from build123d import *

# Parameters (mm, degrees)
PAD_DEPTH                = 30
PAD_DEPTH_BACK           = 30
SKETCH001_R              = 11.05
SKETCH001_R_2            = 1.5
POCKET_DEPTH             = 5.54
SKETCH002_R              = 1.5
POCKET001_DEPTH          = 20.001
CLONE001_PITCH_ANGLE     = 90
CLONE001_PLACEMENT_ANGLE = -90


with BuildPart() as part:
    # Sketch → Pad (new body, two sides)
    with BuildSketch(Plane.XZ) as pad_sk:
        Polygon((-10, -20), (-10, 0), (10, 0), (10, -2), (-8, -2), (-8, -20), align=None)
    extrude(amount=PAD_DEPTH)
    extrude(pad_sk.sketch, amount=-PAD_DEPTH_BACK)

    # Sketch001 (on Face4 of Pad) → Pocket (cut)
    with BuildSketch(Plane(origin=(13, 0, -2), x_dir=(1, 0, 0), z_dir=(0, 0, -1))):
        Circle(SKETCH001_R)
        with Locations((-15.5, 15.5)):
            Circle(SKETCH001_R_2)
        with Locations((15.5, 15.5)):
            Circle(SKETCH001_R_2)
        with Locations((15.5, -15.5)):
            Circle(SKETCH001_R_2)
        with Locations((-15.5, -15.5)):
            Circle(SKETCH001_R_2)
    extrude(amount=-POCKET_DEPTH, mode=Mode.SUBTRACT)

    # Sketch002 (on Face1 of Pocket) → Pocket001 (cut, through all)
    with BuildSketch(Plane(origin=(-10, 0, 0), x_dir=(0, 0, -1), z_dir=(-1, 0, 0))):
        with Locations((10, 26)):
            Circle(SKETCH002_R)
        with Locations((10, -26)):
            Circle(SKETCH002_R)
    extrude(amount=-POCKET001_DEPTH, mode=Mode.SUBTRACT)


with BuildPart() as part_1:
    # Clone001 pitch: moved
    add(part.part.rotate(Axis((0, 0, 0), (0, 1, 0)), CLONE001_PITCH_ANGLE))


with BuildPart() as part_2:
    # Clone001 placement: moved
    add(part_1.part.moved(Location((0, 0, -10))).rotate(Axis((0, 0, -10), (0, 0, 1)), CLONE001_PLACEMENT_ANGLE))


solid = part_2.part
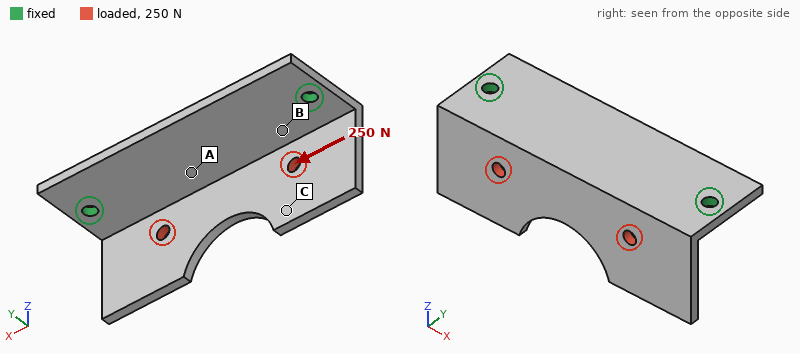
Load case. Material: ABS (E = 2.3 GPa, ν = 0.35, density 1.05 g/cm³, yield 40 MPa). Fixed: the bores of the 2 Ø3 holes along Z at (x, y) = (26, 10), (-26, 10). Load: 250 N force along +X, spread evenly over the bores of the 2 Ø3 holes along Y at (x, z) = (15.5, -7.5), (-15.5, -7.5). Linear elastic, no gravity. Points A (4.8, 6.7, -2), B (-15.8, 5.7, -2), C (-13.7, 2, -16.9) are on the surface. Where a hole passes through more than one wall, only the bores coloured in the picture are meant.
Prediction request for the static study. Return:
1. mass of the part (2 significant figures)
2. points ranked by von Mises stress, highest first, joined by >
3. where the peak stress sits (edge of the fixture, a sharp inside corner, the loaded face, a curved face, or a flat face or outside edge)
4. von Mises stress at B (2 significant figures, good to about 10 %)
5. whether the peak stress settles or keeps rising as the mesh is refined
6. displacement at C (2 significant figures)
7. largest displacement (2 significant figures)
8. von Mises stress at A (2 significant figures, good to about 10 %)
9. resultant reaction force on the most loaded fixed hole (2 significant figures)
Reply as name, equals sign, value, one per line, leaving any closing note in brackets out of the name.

mass of the part = 4.5 g
points ranked by von Mises stress, highest first, joined by > = B > A > C
where the peak stress sits = edge of the fixture
von Mises stress at B = 8.6 MPa
whether the peak stress settles or keeps rising as the mesh is refined = keeps rising
displacement at C = 0.36 mm
largest displacement = 0.66 mm
von Mises stress at A = 5.2 MPa
resultant reaction force on the most loaded fixed hole = 140 N
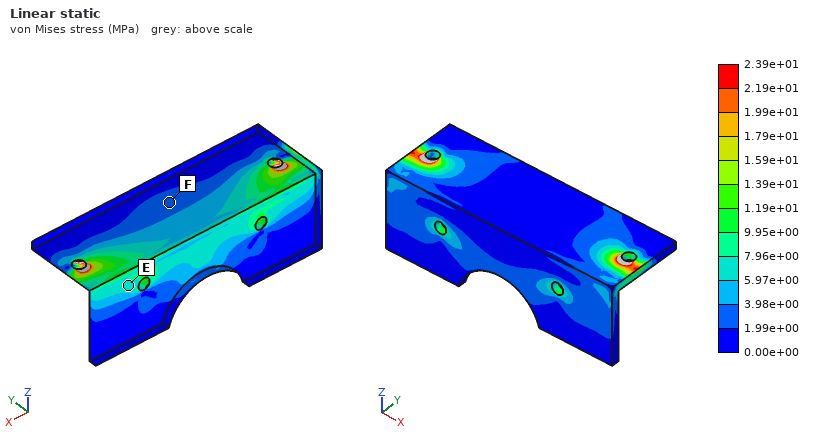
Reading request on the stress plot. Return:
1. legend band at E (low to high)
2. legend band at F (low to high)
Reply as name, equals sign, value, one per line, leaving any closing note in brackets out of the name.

legend band at E = 5.97e+00 to 7.96e+00 MPa
legend band at F = 1.99e+00 to 3.98e+00 MPa
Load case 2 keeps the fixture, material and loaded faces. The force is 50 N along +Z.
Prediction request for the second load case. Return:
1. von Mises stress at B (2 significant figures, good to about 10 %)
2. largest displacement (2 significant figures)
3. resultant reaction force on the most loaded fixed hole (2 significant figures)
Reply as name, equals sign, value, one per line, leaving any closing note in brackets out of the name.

von Mises stress at B = 3.7 MPa
largest displacement = 0.75 mm
resultant reaction force on the most loaded fixed hole = 27 N
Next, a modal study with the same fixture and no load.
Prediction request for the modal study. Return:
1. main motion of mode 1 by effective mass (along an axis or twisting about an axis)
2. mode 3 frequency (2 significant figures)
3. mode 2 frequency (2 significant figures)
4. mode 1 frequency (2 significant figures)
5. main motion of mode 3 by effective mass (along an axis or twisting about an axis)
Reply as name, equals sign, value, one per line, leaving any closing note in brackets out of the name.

main motion of mode 1 by effective mass = along Y
mode 3 frequency = 1500 Hz
mode 2 frequency = 1000 Hz
mode 1 frequency = 710 Hz
main motion of mode 3 by effective mass = along Z
